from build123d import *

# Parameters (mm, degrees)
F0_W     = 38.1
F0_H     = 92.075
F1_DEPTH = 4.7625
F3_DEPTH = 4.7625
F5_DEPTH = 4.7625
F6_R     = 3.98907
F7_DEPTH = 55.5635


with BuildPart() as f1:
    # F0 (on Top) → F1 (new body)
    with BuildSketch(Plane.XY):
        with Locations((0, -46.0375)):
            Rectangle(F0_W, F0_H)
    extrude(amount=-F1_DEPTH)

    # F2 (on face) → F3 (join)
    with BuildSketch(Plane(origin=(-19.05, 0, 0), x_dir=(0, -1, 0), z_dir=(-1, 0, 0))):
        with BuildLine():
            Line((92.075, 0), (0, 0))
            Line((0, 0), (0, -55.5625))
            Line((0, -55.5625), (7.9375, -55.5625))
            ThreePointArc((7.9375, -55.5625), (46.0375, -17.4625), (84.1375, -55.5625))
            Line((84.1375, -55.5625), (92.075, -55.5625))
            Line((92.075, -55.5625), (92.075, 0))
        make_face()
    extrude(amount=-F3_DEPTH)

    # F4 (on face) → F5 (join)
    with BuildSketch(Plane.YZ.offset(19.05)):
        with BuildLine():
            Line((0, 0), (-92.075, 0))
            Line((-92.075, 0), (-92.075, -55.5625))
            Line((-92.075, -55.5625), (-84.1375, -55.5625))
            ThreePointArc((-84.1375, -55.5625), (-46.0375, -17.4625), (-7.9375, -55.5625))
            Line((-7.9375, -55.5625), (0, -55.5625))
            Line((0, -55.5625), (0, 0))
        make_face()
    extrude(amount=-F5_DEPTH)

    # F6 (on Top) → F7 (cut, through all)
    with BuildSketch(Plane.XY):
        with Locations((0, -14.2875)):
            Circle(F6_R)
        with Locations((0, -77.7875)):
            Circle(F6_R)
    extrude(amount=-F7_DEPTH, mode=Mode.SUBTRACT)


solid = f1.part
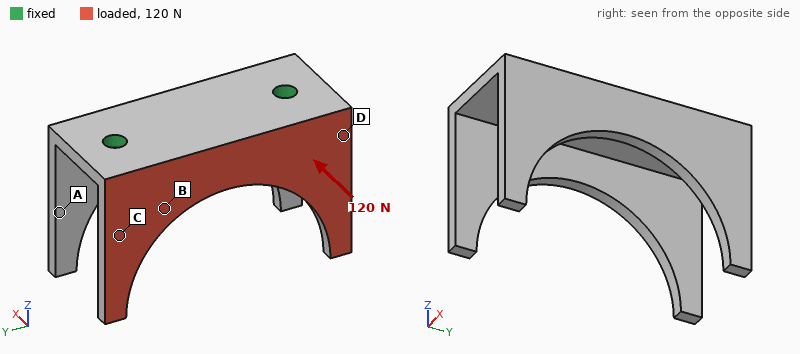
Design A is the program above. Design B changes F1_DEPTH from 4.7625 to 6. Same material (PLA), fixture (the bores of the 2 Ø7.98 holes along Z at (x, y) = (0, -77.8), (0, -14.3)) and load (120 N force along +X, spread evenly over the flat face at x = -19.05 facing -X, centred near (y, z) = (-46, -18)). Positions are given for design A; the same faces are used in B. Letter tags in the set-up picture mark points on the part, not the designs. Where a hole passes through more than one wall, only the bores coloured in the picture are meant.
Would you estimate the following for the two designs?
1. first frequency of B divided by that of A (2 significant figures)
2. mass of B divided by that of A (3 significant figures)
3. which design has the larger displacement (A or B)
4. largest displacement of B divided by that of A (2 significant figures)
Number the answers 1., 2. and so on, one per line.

1. 1.2
2. 1.08
3. A
4. 0.72
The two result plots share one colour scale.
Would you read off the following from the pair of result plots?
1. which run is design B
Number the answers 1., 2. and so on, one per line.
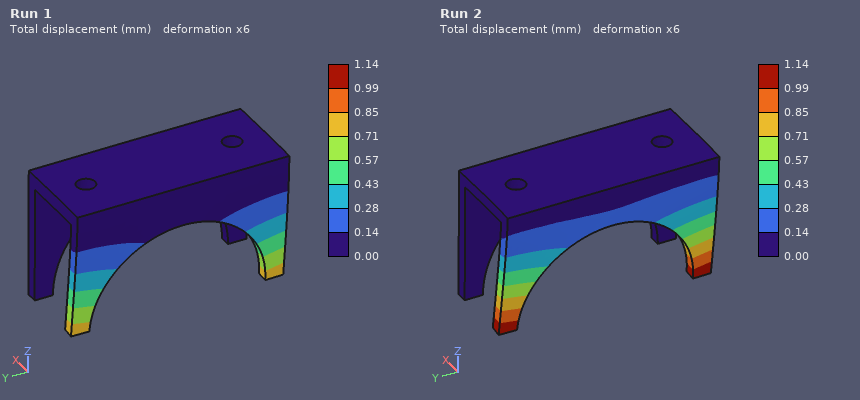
1. Run 1
